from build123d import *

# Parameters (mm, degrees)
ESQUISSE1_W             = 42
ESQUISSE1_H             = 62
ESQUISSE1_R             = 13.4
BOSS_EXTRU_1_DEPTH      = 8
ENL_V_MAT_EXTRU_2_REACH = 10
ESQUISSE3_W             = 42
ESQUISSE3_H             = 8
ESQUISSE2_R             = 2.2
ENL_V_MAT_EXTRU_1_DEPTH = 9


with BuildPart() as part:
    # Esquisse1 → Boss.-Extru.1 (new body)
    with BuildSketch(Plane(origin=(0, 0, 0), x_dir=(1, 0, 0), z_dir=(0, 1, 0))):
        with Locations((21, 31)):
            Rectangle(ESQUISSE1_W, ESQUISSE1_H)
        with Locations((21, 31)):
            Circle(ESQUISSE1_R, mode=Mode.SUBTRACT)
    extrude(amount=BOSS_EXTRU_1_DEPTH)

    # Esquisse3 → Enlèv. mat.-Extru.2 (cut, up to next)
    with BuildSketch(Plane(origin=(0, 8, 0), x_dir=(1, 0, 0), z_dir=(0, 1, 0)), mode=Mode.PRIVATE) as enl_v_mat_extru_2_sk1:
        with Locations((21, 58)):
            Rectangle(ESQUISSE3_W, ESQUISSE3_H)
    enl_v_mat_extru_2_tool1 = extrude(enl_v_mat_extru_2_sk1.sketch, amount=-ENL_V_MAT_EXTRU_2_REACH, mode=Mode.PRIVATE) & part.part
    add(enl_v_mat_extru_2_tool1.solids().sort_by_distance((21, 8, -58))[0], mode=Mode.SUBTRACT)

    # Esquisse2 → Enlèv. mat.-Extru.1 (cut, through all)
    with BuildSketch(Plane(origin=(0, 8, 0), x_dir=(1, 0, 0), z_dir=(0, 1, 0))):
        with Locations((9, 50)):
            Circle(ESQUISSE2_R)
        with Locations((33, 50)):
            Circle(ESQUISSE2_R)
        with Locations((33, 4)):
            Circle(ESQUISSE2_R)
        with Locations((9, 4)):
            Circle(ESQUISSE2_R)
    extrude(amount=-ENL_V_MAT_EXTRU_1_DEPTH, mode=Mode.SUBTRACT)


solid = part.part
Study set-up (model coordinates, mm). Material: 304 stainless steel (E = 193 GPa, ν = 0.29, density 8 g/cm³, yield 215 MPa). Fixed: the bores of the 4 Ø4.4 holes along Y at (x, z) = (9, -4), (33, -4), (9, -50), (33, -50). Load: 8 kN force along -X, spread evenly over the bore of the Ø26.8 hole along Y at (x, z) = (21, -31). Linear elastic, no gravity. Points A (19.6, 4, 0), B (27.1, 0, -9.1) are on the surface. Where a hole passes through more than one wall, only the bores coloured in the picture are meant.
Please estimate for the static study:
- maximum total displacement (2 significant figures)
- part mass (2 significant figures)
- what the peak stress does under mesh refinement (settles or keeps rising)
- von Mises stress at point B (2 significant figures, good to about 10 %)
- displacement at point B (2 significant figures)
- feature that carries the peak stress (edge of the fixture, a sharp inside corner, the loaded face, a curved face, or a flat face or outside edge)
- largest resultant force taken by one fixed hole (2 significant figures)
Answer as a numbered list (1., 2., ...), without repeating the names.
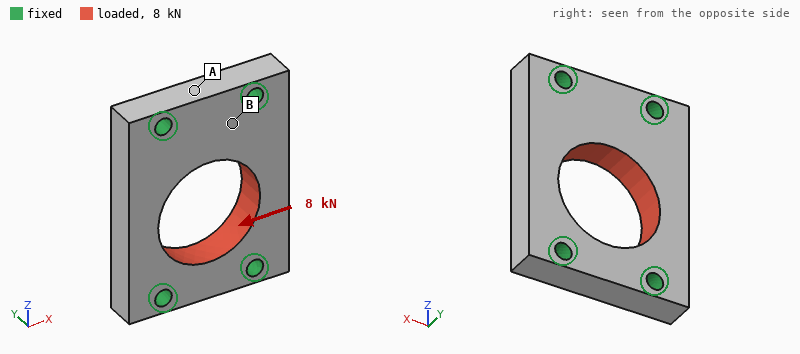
1. 6.0 µm
2. 110 g
3. keeps rising
4. 30 MPa
5. 1.2 µm
6. edge of the fixture
7. 2.1 kN
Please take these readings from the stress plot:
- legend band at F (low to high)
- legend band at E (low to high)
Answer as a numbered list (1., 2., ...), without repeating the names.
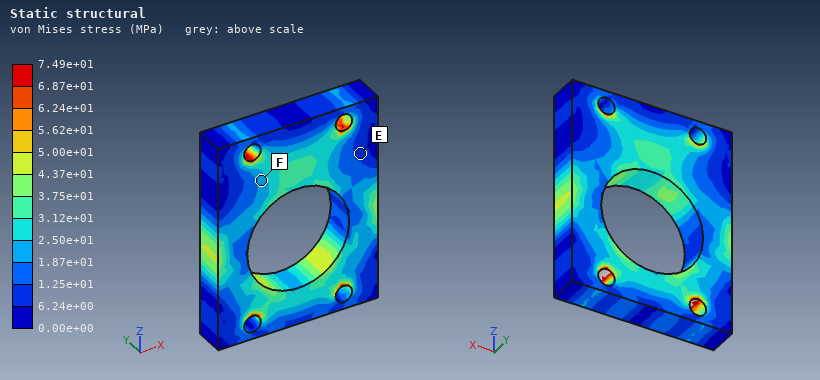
1. 1.87e+01 to 2.50e+01 MPa
2. 6.24e+00 to 1.25e+01 MPa
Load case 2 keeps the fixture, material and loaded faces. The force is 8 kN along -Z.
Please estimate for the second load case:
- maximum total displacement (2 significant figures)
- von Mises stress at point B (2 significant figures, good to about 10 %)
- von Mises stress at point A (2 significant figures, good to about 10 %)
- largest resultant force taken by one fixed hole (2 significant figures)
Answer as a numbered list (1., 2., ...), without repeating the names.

1. 1.7 µm
2. 13 MPa
3. 8.9 MPa
4. 2.2 kN
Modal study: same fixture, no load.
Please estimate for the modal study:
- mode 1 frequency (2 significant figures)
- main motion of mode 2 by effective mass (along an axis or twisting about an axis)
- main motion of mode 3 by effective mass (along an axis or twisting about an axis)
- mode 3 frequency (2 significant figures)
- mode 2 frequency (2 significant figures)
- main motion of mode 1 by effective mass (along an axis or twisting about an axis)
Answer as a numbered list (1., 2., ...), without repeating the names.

1. 17 kHz
2. twisting about Z
3. along X
4. 29 kHz
5. 18 kHz
6. along Y
